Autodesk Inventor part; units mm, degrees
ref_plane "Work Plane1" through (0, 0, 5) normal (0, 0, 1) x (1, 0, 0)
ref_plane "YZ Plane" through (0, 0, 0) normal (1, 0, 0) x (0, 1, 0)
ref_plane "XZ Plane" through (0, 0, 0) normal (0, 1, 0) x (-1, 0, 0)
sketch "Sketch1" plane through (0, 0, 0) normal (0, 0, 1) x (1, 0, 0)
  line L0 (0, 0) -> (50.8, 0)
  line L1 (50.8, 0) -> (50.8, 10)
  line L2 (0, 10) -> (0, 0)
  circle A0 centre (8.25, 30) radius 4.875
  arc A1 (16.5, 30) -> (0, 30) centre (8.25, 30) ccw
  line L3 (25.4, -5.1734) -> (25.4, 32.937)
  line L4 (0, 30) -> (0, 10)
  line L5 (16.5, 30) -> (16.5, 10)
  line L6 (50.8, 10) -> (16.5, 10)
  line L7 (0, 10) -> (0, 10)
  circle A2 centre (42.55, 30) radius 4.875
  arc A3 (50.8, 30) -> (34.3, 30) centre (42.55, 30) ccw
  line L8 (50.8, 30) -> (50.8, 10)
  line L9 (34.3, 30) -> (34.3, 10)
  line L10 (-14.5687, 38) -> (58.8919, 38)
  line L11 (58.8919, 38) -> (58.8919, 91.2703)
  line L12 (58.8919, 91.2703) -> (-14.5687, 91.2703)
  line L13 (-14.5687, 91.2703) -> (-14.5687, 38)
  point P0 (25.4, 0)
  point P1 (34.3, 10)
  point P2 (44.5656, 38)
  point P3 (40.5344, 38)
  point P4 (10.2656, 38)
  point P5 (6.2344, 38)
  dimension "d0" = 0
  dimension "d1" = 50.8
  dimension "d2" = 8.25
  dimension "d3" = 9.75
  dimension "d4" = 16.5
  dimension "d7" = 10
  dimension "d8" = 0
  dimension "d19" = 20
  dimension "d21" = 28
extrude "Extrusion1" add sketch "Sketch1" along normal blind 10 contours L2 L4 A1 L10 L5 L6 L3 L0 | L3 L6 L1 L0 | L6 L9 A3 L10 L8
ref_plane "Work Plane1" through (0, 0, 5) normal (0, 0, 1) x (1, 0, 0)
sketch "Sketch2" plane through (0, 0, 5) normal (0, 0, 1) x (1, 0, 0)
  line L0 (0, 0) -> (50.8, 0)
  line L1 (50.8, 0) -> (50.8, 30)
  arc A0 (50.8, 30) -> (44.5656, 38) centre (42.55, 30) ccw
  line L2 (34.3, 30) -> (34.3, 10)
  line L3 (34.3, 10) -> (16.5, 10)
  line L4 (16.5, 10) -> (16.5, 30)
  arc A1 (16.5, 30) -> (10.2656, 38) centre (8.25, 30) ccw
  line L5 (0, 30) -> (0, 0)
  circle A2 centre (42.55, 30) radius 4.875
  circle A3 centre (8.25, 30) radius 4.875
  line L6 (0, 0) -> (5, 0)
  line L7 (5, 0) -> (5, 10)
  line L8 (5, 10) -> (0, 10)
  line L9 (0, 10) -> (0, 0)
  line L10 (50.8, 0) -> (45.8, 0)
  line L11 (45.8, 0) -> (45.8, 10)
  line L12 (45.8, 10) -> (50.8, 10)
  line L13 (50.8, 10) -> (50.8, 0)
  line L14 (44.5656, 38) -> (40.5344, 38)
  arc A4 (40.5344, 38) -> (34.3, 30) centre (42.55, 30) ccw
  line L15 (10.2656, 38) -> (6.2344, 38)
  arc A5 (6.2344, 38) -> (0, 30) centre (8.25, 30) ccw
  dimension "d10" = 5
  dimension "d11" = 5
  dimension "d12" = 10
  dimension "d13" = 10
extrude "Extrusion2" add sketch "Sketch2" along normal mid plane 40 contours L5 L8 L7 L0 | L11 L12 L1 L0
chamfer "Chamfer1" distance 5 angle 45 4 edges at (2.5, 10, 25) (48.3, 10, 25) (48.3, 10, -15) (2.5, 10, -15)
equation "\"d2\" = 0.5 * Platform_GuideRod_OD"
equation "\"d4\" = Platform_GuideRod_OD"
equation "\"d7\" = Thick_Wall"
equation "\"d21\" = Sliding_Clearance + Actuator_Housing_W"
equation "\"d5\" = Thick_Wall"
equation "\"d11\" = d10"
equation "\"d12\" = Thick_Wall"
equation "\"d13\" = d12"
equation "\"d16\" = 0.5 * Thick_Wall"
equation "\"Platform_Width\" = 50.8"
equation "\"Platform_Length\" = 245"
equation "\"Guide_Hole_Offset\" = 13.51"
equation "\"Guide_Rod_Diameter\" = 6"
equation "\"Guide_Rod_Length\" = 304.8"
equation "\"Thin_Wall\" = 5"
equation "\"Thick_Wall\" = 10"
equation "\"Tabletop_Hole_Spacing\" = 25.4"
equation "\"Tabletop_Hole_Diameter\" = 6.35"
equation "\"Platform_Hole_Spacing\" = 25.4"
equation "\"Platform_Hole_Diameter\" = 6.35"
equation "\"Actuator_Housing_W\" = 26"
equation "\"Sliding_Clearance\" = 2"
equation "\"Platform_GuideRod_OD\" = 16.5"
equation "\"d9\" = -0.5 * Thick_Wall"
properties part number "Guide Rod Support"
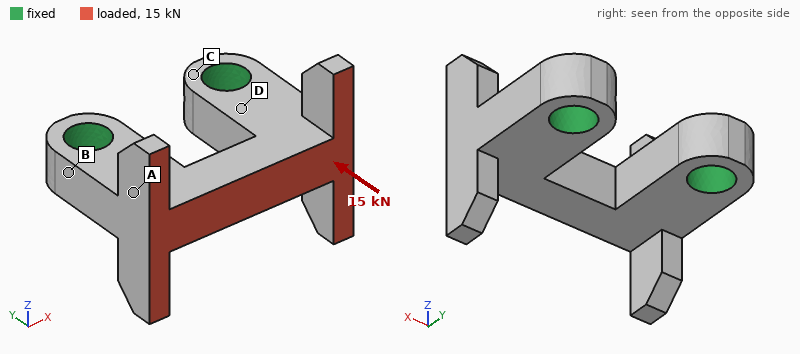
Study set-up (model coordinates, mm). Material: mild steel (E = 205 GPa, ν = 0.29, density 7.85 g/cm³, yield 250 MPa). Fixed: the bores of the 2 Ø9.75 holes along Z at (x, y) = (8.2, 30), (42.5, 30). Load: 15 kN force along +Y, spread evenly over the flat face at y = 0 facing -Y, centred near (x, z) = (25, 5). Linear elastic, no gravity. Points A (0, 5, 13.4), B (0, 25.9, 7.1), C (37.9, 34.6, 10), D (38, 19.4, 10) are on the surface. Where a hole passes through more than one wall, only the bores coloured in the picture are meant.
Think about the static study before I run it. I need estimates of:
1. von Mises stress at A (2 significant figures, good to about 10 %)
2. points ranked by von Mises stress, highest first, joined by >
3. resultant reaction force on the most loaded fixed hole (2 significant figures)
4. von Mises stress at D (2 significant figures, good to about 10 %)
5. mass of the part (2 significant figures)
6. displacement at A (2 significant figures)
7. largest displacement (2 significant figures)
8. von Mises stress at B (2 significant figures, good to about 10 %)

53 MPa
A > D > B > C
7.5 kN
44 MPa
120 g
8.3 µm
23 µm
29 MPa
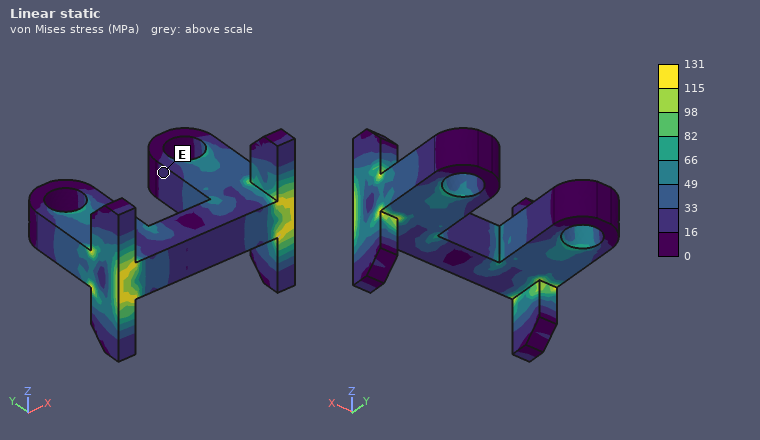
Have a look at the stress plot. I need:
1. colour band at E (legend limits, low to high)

16 to 33 MPa
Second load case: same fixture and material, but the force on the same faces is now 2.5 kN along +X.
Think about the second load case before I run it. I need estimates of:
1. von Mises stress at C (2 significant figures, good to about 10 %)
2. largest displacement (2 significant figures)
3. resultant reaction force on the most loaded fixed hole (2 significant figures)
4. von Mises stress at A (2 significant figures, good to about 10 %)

4.7 MPa
19 µm
1.5 kN
30 MPa
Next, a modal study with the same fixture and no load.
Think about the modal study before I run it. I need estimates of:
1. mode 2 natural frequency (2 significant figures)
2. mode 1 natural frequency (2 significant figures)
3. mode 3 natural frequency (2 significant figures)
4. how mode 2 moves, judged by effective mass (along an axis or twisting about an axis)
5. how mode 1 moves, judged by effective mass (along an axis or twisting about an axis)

8000 Hz
6600 Hz
11 kHz
twisting about Y
along Z
